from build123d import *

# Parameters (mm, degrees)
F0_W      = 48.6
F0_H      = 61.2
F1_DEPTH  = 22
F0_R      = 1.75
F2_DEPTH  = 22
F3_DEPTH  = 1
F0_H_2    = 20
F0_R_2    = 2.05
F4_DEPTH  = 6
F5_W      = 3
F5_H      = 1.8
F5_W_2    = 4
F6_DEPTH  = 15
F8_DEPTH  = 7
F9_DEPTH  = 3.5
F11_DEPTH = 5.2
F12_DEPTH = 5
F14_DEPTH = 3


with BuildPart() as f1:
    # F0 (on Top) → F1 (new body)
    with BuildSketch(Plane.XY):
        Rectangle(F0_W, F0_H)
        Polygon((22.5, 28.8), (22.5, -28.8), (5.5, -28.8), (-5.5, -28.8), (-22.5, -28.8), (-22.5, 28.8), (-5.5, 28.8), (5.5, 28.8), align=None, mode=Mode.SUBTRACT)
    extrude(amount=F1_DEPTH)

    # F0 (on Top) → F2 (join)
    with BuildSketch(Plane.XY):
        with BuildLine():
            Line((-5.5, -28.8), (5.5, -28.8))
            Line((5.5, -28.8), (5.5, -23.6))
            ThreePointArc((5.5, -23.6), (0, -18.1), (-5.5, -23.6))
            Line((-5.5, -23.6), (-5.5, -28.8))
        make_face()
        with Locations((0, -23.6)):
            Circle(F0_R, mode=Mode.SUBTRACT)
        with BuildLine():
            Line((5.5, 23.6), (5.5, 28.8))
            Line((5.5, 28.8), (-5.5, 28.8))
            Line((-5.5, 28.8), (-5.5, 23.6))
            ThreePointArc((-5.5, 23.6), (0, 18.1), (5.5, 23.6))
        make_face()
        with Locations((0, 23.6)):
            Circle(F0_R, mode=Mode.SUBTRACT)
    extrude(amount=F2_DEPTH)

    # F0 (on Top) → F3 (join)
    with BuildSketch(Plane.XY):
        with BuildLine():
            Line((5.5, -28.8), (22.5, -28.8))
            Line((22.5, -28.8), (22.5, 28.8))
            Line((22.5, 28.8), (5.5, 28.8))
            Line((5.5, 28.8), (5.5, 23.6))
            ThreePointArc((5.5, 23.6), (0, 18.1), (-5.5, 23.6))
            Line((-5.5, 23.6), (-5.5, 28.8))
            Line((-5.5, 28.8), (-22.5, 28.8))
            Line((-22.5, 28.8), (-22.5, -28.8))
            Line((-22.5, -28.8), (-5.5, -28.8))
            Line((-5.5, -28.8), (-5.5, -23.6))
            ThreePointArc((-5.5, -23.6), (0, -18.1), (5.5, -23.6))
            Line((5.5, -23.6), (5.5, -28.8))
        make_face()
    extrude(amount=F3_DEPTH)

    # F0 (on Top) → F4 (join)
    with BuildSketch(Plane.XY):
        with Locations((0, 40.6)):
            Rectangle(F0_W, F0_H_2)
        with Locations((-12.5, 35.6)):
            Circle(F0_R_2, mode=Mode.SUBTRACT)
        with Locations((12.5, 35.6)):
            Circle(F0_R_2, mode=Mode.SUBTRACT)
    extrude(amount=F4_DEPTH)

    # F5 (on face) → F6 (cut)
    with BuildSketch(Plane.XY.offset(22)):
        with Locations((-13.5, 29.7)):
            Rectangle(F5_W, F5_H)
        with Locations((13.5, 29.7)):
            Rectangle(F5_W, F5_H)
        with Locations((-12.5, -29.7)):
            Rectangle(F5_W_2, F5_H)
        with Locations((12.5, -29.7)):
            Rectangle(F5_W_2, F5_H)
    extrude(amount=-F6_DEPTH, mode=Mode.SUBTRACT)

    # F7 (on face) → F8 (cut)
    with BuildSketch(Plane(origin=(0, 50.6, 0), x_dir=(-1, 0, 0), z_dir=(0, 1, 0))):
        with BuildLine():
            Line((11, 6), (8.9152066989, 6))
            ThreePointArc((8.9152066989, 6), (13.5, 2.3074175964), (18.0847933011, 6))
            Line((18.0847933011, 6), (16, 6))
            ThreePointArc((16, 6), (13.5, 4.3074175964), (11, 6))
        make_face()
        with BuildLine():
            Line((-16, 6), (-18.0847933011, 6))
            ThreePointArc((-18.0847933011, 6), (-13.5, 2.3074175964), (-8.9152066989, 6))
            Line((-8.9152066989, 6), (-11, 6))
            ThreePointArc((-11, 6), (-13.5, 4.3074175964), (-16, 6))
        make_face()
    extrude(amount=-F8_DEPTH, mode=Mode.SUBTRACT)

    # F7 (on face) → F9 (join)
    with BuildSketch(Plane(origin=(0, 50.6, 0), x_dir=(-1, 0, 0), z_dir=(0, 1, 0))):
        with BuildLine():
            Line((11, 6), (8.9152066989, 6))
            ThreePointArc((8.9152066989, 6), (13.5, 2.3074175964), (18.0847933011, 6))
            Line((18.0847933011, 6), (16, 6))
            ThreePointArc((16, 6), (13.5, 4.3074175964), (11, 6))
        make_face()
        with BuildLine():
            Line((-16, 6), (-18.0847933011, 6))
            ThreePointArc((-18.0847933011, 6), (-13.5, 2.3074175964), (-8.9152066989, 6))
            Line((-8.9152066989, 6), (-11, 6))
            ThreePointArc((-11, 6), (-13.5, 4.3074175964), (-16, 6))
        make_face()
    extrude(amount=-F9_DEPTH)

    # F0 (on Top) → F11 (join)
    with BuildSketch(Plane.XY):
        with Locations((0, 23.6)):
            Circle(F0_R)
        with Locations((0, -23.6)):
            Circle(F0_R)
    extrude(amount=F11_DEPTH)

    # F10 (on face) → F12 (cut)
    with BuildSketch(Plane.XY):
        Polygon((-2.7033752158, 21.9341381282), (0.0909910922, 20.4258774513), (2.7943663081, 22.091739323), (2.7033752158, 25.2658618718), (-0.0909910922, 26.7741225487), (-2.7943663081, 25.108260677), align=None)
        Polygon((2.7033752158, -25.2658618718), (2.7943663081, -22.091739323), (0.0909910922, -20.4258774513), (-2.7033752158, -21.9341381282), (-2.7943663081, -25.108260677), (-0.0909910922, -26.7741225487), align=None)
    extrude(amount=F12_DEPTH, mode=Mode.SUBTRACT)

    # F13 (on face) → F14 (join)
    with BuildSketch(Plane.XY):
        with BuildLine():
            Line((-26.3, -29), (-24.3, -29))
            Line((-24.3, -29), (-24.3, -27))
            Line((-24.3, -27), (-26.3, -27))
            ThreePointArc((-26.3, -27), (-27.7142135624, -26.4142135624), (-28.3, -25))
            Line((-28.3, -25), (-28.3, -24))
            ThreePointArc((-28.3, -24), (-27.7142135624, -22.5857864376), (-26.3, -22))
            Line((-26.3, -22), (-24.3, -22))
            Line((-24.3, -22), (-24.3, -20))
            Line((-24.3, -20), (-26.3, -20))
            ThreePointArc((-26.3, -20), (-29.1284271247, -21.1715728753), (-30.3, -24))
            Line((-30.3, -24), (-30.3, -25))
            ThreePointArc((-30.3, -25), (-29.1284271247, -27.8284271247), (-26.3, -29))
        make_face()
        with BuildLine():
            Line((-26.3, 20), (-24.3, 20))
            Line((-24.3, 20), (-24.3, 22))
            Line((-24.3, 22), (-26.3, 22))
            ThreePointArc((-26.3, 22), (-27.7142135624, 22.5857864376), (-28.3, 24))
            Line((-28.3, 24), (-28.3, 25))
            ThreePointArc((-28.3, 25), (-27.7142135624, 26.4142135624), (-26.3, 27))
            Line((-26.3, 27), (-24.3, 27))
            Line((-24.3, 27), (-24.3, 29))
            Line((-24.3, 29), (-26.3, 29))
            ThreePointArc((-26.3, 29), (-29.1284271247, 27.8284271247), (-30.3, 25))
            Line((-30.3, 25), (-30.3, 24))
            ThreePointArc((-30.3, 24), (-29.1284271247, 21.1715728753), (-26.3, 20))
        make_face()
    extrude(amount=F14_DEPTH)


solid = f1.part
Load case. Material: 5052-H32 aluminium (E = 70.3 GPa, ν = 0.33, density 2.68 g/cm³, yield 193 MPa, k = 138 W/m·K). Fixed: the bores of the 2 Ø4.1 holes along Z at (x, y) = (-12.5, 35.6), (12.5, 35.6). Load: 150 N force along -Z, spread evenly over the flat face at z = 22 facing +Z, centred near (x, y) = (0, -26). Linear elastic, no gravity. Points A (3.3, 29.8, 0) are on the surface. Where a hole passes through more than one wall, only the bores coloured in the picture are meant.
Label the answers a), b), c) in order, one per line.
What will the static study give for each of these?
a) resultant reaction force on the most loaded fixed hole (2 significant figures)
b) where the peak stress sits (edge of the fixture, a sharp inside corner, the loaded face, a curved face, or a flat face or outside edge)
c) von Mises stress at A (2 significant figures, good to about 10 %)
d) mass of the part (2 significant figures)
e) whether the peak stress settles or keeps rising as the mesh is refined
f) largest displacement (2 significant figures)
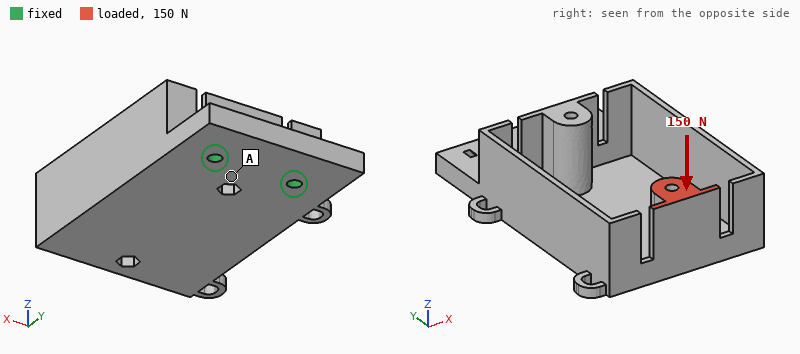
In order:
a) 110 N
b) a sharp inside corner
c) 9.1 MPa
d) 54 g
e) keeps rising
f) 0.37 mm
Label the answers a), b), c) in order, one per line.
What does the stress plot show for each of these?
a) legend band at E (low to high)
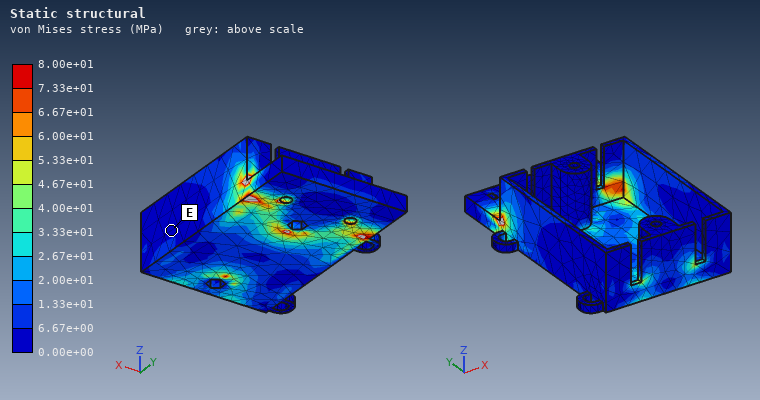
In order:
a) 0.00e+00 to 6.67e+00 MPa
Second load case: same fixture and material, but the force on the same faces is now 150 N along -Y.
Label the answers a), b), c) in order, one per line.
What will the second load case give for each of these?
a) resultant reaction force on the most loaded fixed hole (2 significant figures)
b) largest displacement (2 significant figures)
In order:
a) 82 N
b) 0.46 mm
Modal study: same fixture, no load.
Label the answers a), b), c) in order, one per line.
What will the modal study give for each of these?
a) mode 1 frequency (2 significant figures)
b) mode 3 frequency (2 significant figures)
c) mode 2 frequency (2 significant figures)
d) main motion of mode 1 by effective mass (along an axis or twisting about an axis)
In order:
a) 800 Hz
b) 1800 Hz
c) 1000 Hz
d) along Z
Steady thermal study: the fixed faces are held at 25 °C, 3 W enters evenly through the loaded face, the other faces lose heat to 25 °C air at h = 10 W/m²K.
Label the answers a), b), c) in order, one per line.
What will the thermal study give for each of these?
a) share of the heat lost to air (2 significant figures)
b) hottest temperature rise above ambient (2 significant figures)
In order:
a) 27 %
b) 14 K
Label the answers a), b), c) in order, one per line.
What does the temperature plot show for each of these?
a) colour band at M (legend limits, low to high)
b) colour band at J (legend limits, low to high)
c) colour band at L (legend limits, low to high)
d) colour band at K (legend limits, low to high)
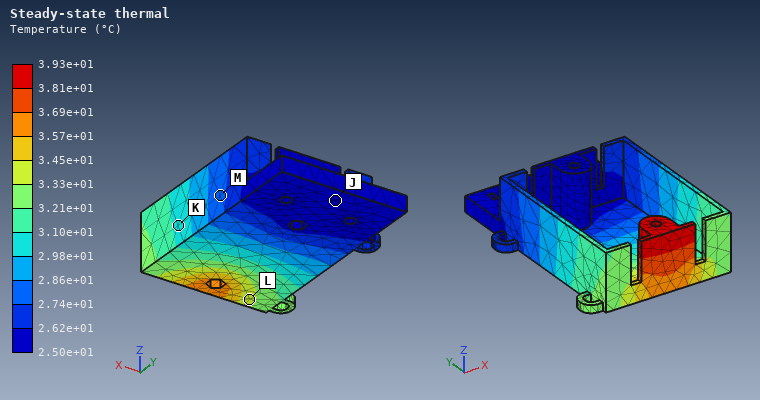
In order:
a) 2.74e+01 to 2.86e+01 °C
b) 2.50e+01 to 2.62e+01 °C
c) 3.33e+01 to 3.45e+01 °C
d) 2.98e+01 to 3.10e+01 °C
